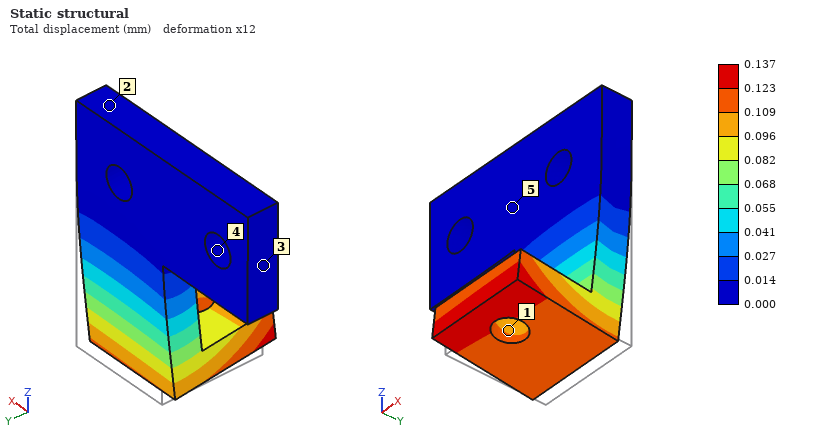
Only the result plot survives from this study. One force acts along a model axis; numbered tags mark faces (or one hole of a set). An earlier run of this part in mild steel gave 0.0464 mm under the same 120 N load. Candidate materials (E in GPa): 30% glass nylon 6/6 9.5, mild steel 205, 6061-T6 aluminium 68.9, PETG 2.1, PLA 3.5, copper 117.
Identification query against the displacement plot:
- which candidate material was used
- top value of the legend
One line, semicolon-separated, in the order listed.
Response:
6061-T6 aluminium; 0.137 mm
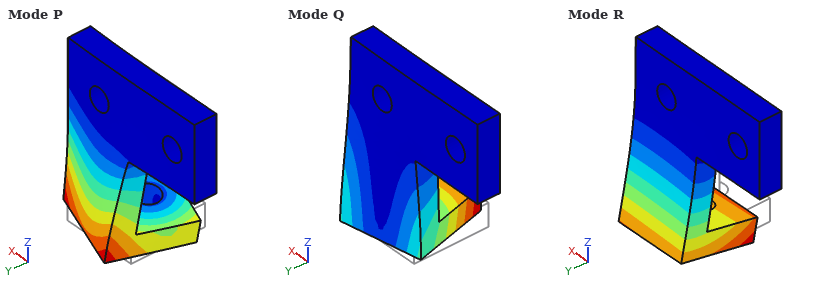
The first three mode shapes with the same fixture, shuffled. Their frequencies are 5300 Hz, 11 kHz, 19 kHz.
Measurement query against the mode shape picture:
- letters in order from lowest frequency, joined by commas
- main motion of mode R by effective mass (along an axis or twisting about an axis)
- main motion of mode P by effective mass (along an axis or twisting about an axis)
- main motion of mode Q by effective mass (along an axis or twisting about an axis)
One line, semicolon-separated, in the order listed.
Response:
R, Q, P; along Y; along X; along X
